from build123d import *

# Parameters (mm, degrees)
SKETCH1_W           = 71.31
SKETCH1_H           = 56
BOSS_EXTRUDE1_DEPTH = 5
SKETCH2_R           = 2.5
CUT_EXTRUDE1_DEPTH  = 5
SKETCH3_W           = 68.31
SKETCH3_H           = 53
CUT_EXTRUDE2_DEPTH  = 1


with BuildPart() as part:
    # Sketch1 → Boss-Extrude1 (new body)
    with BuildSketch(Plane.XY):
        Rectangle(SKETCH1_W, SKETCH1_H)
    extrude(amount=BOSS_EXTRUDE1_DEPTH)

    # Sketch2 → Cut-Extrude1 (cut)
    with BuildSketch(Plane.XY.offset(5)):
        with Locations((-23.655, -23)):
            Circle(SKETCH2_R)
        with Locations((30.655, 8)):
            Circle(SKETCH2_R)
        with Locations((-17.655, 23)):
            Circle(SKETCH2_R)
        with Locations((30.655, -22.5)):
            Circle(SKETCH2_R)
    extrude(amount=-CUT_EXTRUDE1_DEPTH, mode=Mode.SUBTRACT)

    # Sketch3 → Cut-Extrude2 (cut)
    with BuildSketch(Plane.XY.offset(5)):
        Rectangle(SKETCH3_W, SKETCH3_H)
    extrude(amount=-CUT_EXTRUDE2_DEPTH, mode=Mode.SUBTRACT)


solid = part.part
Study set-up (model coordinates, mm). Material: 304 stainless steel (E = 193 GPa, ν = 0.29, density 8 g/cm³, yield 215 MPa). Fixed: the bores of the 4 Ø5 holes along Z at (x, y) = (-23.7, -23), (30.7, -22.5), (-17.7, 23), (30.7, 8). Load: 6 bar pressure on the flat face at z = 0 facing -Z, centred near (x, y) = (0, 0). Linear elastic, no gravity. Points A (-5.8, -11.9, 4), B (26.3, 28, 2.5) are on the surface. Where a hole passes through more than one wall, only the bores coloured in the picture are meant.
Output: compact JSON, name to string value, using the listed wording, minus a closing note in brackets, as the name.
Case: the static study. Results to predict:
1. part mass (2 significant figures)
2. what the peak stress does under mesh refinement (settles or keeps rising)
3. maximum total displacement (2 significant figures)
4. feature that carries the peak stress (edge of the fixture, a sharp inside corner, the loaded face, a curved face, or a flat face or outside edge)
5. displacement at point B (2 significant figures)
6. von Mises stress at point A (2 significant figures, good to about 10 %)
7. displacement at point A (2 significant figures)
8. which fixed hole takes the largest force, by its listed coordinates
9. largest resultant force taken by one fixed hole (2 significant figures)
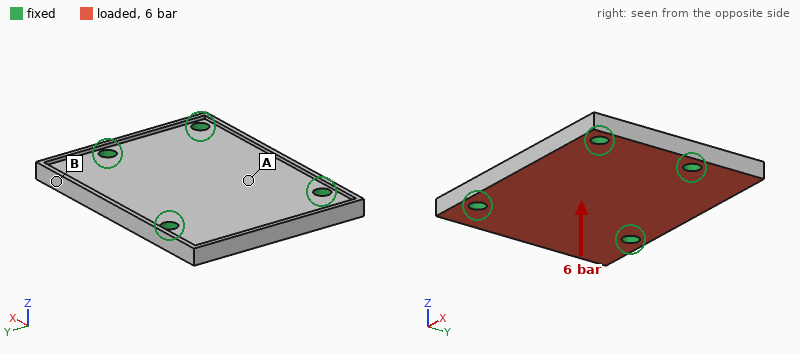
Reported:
{"part mass": "130 g", "what the peak stress does under mesh refinement": "keeps rising", "maximum total displacement": "15 µm", "feature that carries the peak stress": "edge of the fixture", "displacement at point B": "10 µm", "von Mises stress at point A": "18 MPa", "displacement at point A": "13 µm", "which fixed hole takes the largest force, by its listed coordinates": "(-17.7, 23)", "largest resultant force taken by one fixed hole": "720 N"}
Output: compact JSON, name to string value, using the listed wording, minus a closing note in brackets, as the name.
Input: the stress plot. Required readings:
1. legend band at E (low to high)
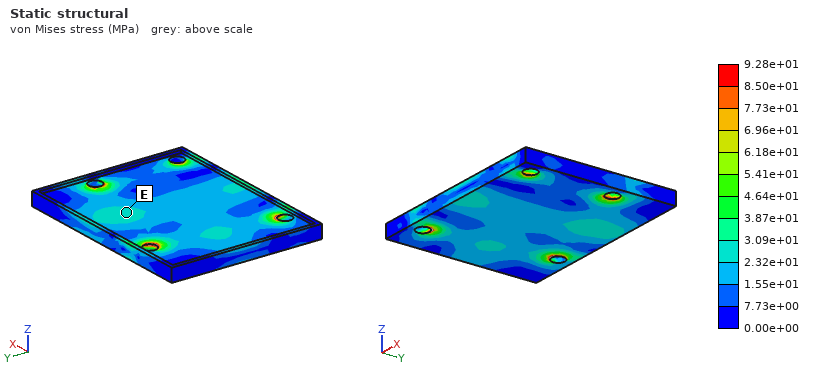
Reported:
{"legend band at E": "2.32e+01 to 3.09e+01 MPa"}
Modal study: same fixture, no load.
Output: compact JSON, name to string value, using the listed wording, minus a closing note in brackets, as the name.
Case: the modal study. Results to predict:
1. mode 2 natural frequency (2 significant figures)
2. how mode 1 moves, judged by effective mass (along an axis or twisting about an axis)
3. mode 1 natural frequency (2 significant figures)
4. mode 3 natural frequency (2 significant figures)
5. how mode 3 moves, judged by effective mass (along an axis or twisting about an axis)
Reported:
{"mode 2 natural frequency": "7300 Hz", "how mode 1 moves, judged by effective mass": "along Z", "mode 1 natural frequency": "6500 Hz", "mode 3 natural frequency": "7900 Hz", "how mode 3 moves, judged by effective mass": "along Z"}
